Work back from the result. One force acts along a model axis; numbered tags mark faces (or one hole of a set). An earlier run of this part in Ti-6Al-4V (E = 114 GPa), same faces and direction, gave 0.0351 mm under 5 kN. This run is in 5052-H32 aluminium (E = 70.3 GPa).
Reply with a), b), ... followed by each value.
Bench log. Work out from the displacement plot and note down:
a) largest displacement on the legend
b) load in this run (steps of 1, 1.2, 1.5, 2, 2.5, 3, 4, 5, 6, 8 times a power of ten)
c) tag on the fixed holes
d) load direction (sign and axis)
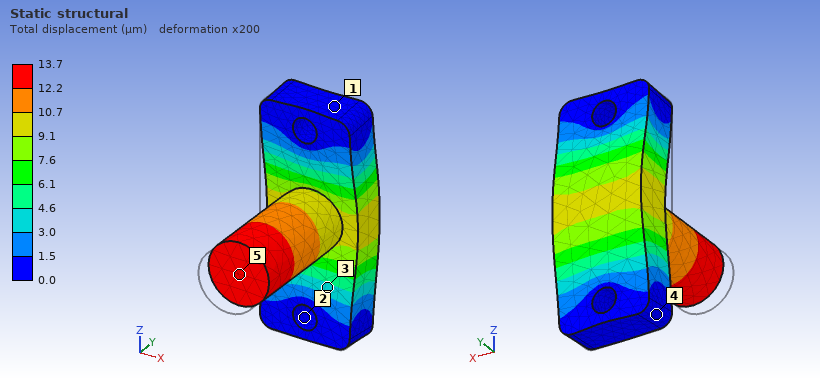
a) 13.7 µm
b) 1.2 kN
c) 2
d) +Y
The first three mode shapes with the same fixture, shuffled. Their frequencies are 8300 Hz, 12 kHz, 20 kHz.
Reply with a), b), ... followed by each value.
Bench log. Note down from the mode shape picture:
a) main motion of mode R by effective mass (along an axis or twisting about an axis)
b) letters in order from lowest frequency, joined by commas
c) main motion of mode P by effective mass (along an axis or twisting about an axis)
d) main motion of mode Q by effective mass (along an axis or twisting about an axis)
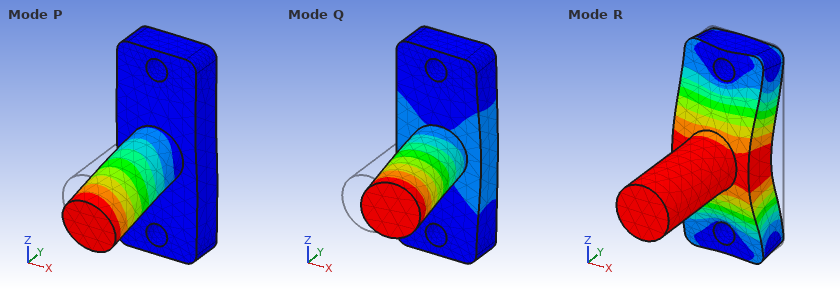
a) along Y
b) Q, P, R
c) along Z
d) along X
